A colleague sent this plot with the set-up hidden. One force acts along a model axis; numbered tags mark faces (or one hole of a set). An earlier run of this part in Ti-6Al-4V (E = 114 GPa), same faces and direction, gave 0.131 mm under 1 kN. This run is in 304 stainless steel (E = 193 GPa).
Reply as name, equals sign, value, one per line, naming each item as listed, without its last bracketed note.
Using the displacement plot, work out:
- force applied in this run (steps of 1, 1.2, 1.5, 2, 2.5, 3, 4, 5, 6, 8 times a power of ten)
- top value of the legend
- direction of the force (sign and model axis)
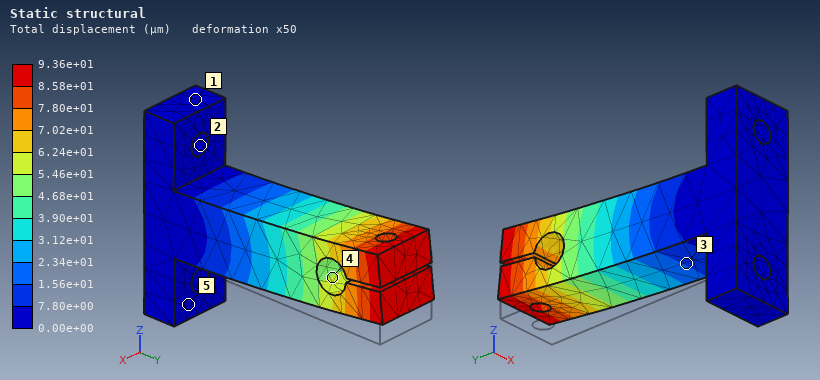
force applied in this run = 1.2 kN
top value of the legend = 9.36e+01 µm
direction of the force = +Z
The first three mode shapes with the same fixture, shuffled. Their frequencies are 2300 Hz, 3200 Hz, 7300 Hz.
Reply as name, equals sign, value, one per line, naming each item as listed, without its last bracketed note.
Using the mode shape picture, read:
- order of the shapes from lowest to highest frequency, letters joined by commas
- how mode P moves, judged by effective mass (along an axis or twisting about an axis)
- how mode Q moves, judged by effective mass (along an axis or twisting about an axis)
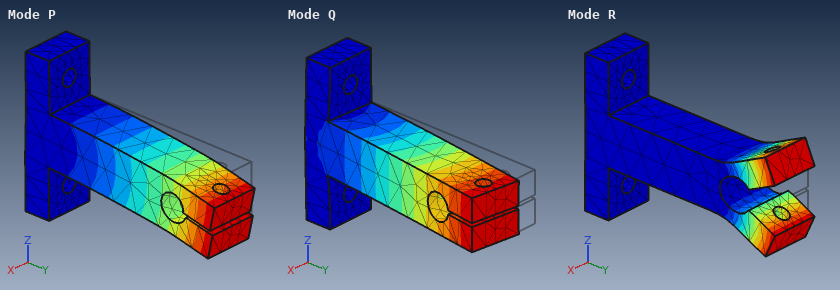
order of the shapes from lowest to highest frequency, letters joined by commas = Q, P, R
how mode P moves, judged by effective mass = along Z
how mode Q moves, judged by effective mass = along X
